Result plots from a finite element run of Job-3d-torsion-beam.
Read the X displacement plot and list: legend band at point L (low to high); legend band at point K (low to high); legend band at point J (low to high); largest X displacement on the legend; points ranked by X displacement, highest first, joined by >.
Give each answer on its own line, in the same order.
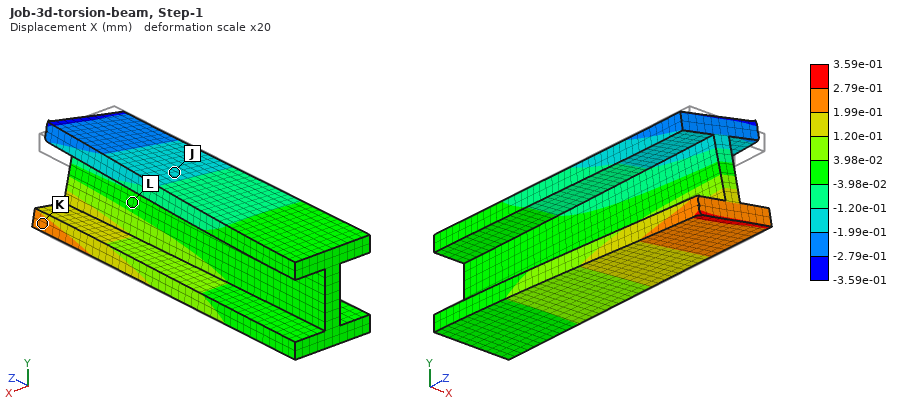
-3.98e-02 to 3.98e-02 mm
1.99e-01 to 2.79e-01 mm
-1.99e-01 to -1.20e-01 mm
3.59e-01 mm
K > L > J
